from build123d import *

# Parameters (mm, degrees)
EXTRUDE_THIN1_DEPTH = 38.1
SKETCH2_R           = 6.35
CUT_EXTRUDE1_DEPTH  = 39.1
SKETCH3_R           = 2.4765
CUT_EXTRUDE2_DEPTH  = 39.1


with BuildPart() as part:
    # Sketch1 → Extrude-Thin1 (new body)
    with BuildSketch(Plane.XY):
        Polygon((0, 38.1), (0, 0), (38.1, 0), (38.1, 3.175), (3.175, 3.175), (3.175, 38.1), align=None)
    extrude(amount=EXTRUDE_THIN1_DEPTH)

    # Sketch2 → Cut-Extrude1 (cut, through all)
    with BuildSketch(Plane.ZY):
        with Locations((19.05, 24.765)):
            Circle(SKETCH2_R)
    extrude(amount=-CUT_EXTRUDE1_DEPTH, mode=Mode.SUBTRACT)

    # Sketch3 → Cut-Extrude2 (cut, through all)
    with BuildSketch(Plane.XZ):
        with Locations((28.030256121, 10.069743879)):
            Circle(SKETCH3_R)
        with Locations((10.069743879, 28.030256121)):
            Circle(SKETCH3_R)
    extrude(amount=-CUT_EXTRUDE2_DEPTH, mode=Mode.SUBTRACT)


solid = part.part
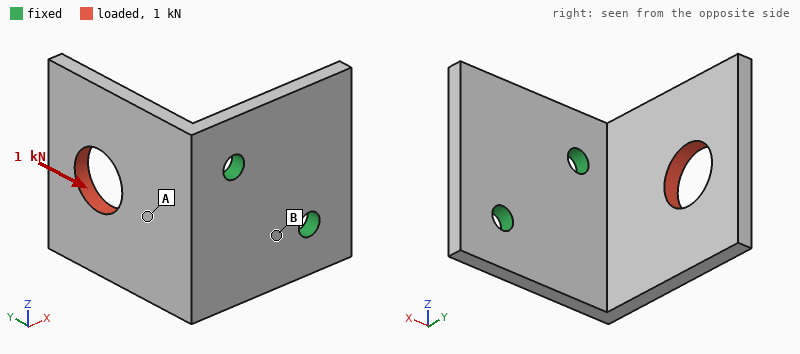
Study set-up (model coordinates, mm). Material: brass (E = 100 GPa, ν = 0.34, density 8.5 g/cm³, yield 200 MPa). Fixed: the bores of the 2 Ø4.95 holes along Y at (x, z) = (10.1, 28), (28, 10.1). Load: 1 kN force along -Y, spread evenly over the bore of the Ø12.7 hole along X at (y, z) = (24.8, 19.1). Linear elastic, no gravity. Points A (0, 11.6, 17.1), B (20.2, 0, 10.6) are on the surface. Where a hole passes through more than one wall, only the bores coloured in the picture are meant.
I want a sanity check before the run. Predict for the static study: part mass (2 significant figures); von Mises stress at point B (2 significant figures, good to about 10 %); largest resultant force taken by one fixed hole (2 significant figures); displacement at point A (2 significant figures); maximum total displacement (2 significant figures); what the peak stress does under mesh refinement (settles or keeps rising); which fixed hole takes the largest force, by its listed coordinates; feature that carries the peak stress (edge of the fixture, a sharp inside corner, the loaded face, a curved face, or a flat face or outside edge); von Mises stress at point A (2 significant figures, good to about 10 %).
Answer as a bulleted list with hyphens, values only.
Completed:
- 71 g
- 60 MPa
- 940 N
- 0.10 mm
- 0.30 mm
- keeps rising
- (10.1, 28)
- edge of the fixture
- 22 MPa
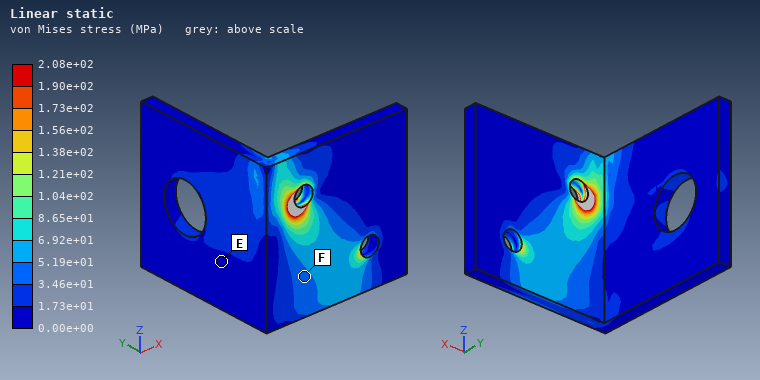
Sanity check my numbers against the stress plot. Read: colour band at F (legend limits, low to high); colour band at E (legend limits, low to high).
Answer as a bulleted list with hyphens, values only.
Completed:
- 3.46e+01 to 5.19e+01 MPa
- 0.00e+00 to 1.73e+01 MPa
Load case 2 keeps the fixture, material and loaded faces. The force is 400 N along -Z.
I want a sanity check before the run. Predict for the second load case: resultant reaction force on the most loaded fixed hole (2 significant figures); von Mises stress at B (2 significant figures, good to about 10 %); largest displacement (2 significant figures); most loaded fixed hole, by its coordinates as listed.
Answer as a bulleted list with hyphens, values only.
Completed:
- 440 N
- 52 MPa
- 0.21 mm
- (10.1, 28)
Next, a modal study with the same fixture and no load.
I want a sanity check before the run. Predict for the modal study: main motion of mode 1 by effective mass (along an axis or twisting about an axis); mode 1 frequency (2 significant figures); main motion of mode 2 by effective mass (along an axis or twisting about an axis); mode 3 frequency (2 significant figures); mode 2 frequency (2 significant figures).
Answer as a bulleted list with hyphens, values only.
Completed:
- along X
- 980 Hz
- along Z
- 2700 Hz
- 1600 Hz
